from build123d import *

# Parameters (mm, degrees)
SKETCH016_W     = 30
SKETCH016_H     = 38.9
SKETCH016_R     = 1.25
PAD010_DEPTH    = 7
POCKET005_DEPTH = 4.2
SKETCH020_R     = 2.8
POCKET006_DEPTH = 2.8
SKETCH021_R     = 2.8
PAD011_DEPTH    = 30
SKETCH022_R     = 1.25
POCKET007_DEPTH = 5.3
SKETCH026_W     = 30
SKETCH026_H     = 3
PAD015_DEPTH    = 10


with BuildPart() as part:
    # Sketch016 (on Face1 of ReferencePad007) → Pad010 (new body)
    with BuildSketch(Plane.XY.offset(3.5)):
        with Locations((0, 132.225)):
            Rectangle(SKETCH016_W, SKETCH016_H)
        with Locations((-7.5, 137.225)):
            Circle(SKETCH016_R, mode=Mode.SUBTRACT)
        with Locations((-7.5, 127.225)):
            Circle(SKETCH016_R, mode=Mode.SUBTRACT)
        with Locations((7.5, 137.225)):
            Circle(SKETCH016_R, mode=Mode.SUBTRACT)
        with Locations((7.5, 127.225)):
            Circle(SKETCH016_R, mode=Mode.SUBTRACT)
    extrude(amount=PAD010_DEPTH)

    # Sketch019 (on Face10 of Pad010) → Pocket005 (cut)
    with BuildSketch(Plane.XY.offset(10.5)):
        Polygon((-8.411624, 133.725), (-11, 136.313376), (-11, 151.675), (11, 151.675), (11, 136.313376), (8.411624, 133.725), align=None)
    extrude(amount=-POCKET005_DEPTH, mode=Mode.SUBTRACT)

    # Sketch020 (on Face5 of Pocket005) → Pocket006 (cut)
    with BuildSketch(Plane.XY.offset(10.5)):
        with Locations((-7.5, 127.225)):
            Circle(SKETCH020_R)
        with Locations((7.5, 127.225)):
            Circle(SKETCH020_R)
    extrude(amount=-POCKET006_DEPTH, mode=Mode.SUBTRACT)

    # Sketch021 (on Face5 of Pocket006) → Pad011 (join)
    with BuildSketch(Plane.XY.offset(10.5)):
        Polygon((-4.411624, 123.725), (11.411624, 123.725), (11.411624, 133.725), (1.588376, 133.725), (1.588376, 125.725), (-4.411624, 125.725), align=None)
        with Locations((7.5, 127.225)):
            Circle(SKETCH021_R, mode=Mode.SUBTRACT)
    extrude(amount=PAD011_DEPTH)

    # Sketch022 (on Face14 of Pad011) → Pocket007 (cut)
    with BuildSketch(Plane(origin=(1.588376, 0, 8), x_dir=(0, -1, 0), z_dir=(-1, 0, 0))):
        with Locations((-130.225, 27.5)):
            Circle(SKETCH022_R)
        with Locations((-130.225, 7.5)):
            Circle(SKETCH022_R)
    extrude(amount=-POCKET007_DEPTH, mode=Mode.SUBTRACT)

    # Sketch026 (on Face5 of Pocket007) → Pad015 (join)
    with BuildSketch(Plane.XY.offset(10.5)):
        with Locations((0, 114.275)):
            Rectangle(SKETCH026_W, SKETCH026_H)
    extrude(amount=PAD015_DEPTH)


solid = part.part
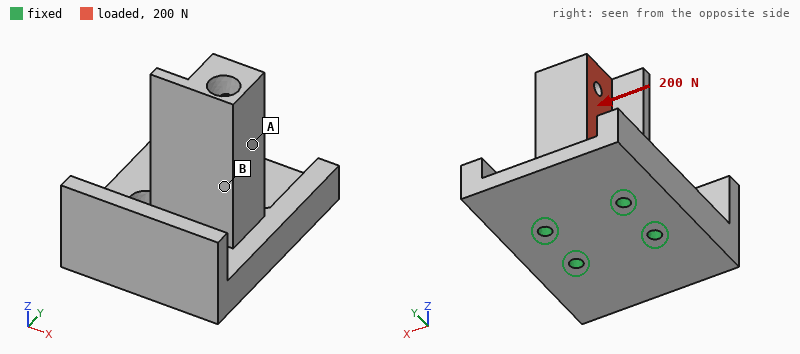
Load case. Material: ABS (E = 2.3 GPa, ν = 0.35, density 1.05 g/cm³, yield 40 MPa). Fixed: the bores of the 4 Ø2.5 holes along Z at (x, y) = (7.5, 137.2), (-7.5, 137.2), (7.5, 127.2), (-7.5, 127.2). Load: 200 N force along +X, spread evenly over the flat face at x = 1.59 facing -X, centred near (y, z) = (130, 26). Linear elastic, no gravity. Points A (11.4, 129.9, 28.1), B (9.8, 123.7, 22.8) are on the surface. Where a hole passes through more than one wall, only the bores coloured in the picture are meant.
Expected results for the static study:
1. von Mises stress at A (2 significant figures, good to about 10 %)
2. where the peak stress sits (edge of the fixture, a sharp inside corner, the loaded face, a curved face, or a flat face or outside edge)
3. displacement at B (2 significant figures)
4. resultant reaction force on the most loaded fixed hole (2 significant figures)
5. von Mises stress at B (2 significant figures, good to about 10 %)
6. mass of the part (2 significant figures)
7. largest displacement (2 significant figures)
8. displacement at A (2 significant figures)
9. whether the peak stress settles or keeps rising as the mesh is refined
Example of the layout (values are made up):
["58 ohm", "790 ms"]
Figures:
["3.4 MPa", "edge of the fixture", "0.23 mm", "230 N", "7.2 MPa", "10 g", "0.61 mm", "0.35 mm", "keeps rising"]
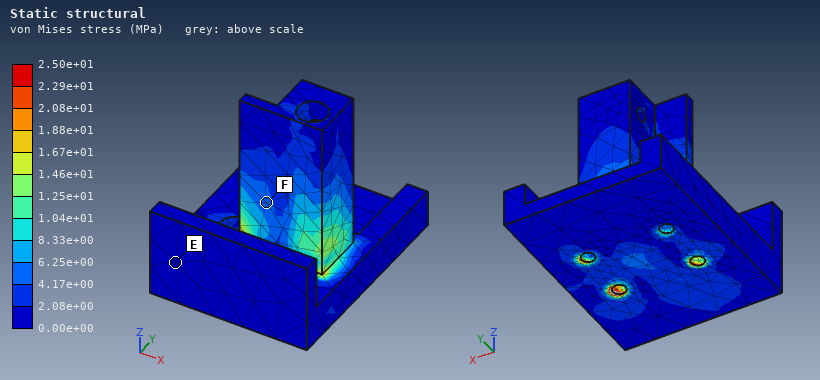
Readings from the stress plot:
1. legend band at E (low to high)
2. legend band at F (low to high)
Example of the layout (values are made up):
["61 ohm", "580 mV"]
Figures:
["0.00e+00 to 2.08e+00 MPa", "4.17e+00 to 6.25e+00 MPa"]
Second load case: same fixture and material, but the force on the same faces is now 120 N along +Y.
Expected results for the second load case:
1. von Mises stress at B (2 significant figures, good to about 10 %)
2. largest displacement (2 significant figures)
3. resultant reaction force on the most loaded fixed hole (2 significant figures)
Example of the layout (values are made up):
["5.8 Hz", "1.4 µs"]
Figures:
["5.8 MPa", "0.66 mm", "130 N"]
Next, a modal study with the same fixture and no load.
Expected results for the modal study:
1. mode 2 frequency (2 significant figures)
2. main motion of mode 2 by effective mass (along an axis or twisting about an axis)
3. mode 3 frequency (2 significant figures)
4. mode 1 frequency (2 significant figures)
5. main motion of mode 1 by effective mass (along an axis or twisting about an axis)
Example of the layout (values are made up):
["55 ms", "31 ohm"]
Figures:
["2400 Hz", "along X", "3400 Hz", "1600 Hz", "along Y"]
